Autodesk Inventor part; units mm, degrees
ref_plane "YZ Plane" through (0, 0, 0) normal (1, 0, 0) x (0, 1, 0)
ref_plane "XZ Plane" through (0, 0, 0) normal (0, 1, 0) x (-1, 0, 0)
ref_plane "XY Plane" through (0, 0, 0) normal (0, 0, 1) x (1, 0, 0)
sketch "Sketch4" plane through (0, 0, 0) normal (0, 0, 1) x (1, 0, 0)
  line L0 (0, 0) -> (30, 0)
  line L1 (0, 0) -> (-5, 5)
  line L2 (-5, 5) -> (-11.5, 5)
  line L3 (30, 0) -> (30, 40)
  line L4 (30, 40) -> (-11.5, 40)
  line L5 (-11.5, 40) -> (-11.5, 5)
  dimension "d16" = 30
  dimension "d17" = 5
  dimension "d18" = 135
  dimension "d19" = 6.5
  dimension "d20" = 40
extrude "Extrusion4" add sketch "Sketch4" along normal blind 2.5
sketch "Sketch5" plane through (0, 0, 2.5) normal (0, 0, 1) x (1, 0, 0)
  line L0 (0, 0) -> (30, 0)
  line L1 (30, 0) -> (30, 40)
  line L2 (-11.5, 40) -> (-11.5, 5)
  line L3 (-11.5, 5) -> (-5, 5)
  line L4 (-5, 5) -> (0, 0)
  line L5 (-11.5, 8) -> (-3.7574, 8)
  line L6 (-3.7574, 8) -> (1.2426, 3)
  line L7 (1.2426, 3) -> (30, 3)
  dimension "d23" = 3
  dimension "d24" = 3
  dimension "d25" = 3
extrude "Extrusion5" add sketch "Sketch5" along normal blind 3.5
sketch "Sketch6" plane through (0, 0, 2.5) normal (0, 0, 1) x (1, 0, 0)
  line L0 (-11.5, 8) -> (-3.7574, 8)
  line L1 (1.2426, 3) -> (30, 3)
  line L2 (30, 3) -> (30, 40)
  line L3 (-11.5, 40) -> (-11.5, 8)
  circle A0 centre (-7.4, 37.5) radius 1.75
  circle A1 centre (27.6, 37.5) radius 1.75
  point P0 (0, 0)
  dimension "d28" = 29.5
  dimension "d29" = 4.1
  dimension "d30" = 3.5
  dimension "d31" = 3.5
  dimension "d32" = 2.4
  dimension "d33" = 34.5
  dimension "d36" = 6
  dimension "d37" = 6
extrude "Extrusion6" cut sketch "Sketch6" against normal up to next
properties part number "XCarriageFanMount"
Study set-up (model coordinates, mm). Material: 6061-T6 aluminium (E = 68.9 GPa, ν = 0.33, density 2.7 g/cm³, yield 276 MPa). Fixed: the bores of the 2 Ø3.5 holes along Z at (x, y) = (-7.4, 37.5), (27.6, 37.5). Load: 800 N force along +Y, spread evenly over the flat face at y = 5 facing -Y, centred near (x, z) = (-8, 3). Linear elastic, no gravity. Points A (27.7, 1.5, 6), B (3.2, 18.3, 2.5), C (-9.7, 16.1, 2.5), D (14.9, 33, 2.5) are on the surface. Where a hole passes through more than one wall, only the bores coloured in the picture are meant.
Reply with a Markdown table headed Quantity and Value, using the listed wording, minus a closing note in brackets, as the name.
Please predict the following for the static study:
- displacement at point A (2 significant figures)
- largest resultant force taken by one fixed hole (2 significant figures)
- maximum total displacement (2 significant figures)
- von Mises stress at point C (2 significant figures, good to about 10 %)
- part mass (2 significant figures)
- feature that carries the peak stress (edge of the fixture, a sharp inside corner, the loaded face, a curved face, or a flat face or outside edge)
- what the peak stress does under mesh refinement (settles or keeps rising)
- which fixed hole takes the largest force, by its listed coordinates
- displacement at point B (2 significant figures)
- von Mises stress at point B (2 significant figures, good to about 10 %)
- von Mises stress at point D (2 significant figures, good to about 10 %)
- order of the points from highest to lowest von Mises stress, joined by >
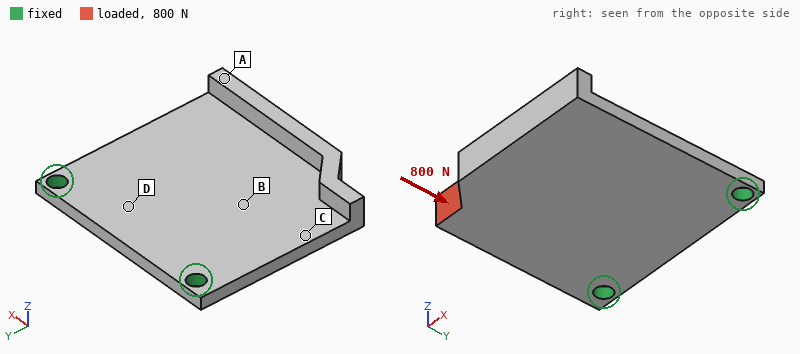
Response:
| Quantity | Value |
|---|---|
| displacement at point A | 0.24 mm |
| largest resultant force taken by one fixed hole | 820 N |
| maximum total displacement | 0.33 mm |
| von Mises stress at point C | 85 MPa |
| part mass | 12 g |
| feature that carries the peak stress | edge of the fixture |
| what the peak stress does under mesh refinement | keeps rising |
| which fixed hole takes the largest force, by its listed coordinates | (-7.4, 37.5) |
| displacement at point B | 0.099 mm |
| von Mises stress at point B | 39 MPa |
| von Mises stress at point D | 21 MPa |
| order of the points from highest to lowest von Mises stress, joined by > | C > B > D > A |
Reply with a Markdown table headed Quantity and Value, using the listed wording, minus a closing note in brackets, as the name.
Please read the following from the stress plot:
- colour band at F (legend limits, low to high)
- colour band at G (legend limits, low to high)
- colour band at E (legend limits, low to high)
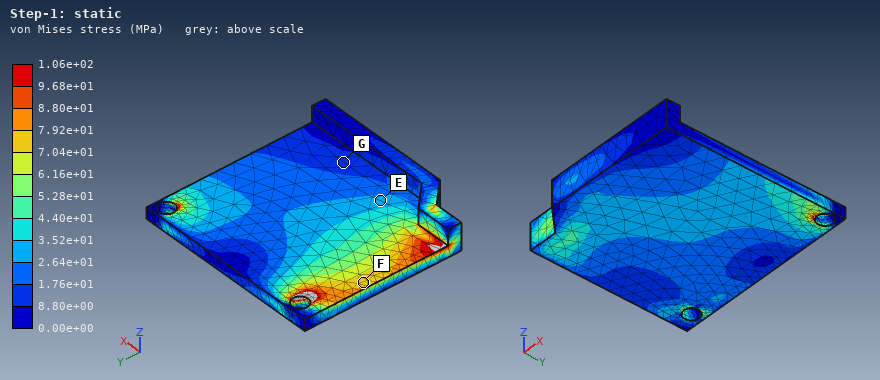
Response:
| Quantity | Value |
|---|---|
| colour band at F | 7.04e+01 to 7.92e+01 MPa |
| colour band at G | 8.80e+00 to 1.76e+01 MPa |
| colour band at E | 2.64e+01 to 3.52e+01 MPa |
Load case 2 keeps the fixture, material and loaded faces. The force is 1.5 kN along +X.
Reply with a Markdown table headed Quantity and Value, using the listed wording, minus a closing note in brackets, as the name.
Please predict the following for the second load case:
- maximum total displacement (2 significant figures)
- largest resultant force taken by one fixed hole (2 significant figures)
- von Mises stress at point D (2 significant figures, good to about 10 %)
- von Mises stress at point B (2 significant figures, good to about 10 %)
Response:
| Quantity | Value |
|---|---|
| maximum total displacement | 0.23 mm |
| largest resultant force taken by one fixed hole | 1.6 kN |
| von Mises stress at point D | 36 MPa |
| von Mises stress at point B | 80 MPa |
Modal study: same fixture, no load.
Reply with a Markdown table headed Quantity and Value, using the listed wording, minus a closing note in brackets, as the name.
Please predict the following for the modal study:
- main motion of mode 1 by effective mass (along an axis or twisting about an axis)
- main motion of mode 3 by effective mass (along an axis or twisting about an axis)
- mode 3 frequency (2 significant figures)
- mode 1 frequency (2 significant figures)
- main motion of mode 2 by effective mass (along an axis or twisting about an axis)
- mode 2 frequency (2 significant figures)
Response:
| Quantity | Value |
|---|---|
| main motion of mode 1 by effective mass | along Z |
| main motion of mode 3 by effective mass | along Z |
| mode 3 frequency | 7300 Hz |
| mode 1 frequency | 1100 Hz |
| main motion of mode 2 by effective mass | twisting about Y |
| mode 2 frequency | 3300 Hz |
